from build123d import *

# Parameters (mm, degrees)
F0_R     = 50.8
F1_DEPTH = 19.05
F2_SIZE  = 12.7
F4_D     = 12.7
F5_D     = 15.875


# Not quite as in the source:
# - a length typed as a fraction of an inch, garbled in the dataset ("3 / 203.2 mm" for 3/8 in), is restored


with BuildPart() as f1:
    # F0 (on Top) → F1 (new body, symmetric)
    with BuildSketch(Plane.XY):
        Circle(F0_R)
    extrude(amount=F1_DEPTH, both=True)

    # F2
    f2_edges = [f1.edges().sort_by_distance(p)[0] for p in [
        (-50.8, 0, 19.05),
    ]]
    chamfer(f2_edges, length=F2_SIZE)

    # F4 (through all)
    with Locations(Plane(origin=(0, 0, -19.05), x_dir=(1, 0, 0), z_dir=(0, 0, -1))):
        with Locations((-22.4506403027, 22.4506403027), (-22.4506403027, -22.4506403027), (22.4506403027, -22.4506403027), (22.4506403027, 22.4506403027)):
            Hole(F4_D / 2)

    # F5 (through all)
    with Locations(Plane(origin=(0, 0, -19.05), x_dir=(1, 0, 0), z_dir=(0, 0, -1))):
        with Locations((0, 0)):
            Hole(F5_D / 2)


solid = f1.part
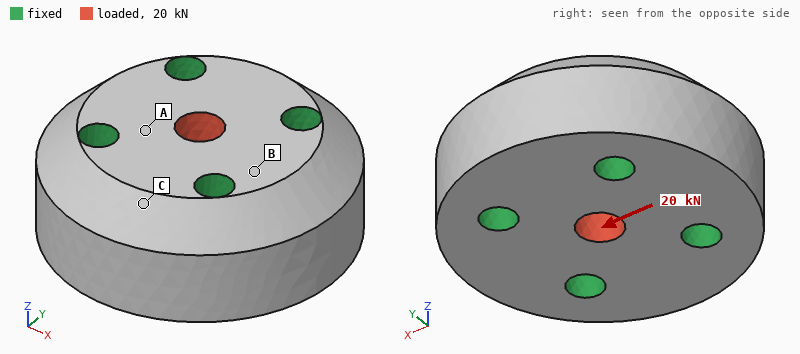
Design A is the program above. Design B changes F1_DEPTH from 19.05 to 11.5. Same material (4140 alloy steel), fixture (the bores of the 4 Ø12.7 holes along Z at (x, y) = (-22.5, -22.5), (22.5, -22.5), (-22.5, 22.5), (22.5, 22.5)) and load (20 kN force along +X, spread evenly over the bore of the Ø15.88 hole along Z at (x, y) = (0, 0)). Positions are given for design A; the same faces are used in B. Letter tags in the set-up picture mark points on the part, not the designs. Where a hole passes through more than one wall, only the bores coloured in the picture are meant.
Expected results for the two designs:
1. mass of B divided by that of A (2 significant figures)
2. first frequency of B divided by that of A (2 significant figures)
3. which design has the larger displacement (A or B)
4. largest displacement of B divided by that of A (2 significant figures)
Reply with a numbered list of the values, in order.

1. 0.57
2. 0.87
3. B
4. 1.6
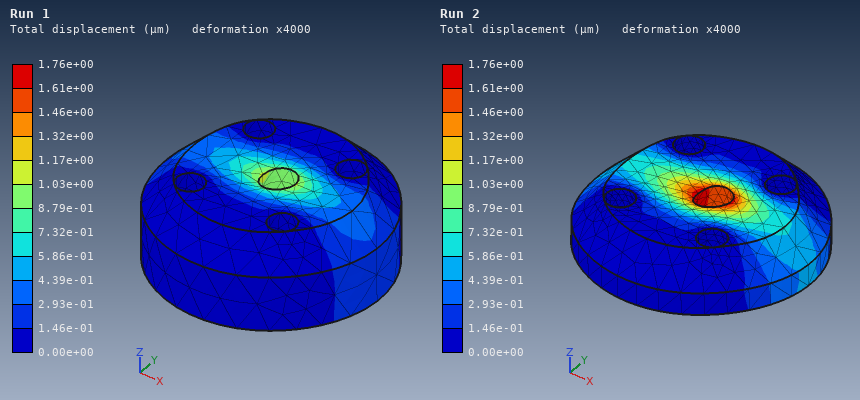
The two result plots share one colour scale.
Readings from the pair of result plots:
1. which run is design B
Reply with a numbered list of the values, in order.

1. Run 2
